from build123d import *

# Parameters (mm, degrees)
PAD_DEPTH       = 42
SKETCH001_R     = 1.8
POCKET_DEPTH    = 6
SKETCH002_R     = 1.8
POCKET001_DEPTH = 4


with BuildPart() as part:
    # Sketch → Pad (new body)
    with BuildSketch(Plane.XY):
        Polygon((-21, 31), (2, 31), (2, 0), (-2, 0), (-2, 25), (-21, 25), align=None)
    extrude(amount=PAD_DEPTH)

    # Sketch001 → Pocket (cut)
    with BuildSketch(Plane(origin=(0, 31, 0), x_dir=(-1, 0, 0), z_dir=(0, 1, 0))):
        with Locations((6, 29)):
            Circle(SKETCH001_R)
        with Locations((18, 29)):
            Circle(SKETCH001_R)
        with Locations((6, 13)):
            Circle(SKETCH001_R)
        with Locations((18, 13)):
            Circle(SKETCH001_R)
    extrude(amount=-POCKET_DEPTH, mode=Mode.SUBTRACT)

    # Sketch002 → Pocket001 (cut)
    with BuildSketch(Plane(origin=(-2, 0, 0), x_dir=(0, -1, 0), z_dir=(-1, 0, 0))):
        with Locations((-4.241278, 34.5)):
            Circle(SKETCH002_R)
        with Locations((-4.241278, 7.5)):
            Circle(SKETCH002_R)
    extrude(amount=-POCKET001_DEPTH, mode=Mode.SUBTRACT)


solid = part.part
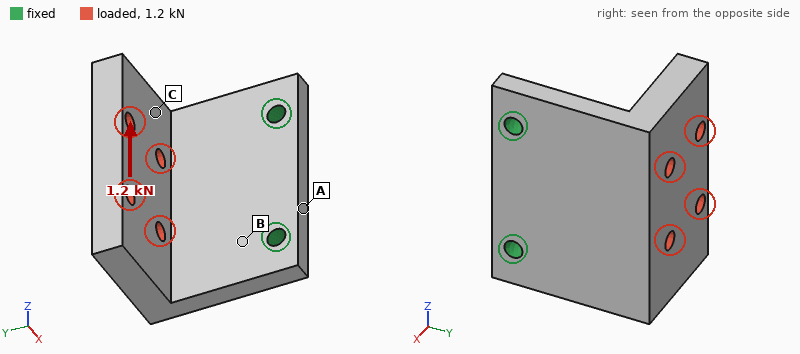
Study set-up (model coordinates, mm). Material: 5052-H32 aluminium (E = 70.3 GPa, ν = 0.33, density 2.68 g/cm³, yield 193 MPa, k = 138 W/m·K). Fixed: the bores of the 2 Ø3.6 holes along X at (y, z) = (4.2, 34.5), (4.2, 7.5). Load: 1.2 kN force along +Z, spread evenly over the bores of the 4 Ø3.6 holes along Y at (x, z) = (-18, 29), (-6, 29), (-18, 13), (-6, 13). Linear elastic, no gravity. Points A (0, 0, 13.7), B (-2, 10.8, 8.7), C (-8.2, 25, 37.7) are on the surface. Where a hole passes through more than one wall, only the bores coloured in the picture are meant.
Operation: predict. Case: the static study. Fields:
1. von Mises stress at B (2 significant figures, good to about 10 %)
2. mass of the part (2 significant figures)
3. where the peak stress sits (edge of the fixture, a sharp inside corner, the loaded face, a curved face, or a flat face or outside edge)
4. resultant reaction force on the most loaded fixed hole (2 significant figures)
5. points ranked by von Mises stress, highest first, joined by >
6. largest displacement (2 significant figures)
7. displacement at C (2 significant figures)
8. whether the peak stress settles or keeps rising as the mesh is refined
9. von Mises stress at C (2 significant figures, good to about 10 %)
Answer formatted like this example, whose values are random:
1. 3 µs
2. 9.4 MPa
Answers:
1. 66 MPa
2. 26 g
3. edge of the fixture
4. 1.2 kN
5. B > C > A
6. 0.17 mm
7. 0.10 mm
8. keeps rising
9. 29 MPa
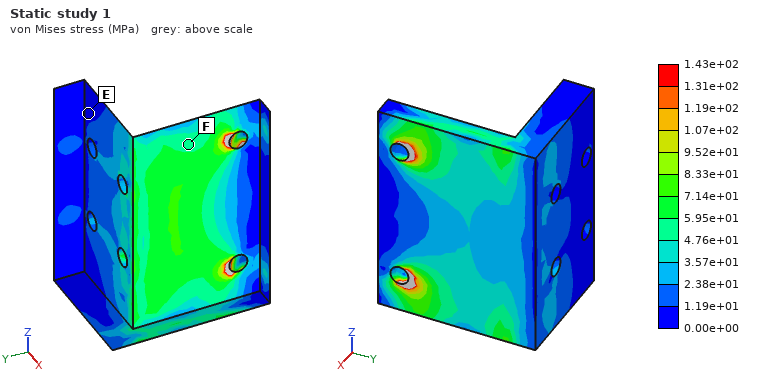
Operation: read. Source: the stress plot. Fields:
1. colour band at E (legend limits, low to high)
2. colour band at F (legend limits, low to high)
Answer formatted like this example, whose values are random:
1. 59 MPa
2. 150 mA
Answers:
1. 0.00e+00 to 1.19e+01 MPa
2. 4.76e+01 to 5.95e+01 MPa
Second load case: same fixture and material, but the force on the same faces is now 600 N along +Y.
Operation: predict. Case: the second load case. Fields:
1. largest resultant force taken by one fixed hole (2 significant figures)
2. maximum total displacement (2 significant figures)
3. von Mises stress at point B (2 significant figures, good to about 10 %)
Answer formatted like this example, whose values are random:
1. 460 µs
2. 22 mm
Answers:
1. 310 N
2. 0.29 mm
3. 72 MPa
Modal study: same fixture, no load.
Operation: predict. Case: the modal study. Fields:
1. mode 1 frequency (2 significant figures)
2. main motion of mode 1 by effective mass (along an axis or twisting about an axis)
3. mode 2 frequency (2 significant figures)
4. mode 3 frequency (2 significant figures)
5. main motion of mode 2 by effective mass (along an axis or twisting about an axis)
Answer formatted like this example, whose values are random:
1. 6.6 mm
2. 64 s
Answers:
1. 1800 Hz
2. along X
3. 3700 Hz
4. 6400 Hz
5. along Z
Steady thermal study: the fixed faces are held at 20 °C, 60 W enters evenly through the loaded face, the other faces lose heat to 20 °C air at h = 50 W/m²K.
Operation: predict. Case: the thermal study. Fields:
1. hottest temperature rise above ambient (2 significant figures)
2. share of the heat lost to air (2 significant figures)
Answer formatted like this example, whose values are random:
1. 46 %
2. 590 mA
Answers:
1. 78 K
2. 18 %
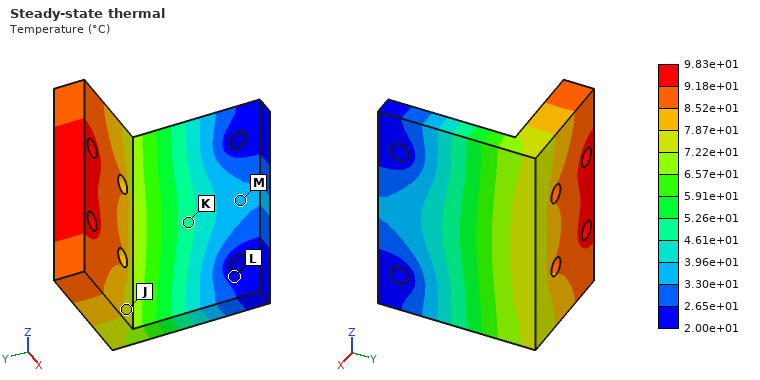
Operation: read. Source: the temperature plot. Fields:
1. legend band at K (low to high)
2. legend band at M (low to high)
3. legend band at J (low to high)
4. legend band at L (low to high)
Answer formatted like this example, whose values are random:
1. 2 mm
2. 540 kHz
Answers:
1. 4.61e+01 to 5.26e+01 °C
2. 3.30e+01 to 3.96e+01 °C
3. 7.22e+01 to 7.87e+01 °C
4. 2.00e+01 to 2.65e+01 °C
